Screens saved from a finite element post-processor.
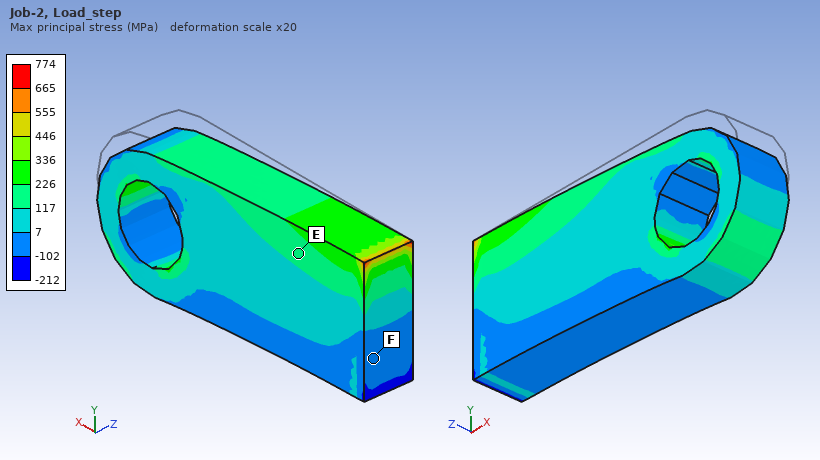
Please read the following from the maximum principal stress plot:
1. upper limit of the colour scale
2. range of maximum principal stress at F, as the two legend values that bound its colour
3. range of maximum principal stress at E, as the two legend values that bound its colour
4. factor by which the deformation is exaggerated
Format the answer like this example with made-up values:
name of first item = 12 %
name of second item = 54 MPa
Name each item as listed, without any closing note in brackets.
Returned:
upper limit of the colour scale = 774 MPa
range of maximum principal stress at F, as the two legend values that bound its colour = -102 to 7 MPa
range of maximum principal stress at E, as the two legend values that bound its colour = 117 to 226 MPa
factor by which the deformation is exaggerated = 20
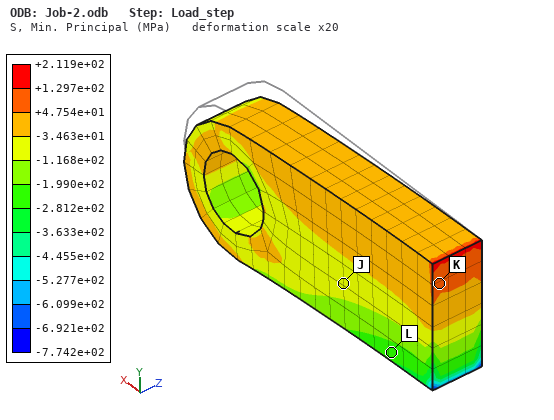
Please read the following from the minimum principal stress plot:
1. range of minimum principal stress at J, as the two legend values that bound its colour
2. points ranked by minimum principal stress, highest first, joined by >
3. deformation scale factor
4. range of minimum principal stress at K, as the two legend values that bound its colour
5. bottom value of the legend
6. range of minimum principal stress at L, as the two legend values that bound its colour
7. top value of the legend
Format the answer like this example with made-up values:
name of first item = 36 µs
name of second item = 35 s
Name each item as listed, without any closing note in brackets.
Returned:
range of minimum principal stress at J, as the two legend values that bound its colour = -1.168e+02 to -3.463e+01 MPa
points ranked by minimum principal stress, highest first, joined by > = K > J > L
deformation scale factor = 20
range of minimum principal stress at K, as the two legend values that bound its colour = +4.754e+01 to +1.297e+02 MPa
bottom value of the legend = -7.742e+02 MPa
range of minimum principal stress at L, as the two legend values that bound its colour = -2.812e+02 to -1.990e+02 MPa
top value of the legend = +2.119e+02 MPa
